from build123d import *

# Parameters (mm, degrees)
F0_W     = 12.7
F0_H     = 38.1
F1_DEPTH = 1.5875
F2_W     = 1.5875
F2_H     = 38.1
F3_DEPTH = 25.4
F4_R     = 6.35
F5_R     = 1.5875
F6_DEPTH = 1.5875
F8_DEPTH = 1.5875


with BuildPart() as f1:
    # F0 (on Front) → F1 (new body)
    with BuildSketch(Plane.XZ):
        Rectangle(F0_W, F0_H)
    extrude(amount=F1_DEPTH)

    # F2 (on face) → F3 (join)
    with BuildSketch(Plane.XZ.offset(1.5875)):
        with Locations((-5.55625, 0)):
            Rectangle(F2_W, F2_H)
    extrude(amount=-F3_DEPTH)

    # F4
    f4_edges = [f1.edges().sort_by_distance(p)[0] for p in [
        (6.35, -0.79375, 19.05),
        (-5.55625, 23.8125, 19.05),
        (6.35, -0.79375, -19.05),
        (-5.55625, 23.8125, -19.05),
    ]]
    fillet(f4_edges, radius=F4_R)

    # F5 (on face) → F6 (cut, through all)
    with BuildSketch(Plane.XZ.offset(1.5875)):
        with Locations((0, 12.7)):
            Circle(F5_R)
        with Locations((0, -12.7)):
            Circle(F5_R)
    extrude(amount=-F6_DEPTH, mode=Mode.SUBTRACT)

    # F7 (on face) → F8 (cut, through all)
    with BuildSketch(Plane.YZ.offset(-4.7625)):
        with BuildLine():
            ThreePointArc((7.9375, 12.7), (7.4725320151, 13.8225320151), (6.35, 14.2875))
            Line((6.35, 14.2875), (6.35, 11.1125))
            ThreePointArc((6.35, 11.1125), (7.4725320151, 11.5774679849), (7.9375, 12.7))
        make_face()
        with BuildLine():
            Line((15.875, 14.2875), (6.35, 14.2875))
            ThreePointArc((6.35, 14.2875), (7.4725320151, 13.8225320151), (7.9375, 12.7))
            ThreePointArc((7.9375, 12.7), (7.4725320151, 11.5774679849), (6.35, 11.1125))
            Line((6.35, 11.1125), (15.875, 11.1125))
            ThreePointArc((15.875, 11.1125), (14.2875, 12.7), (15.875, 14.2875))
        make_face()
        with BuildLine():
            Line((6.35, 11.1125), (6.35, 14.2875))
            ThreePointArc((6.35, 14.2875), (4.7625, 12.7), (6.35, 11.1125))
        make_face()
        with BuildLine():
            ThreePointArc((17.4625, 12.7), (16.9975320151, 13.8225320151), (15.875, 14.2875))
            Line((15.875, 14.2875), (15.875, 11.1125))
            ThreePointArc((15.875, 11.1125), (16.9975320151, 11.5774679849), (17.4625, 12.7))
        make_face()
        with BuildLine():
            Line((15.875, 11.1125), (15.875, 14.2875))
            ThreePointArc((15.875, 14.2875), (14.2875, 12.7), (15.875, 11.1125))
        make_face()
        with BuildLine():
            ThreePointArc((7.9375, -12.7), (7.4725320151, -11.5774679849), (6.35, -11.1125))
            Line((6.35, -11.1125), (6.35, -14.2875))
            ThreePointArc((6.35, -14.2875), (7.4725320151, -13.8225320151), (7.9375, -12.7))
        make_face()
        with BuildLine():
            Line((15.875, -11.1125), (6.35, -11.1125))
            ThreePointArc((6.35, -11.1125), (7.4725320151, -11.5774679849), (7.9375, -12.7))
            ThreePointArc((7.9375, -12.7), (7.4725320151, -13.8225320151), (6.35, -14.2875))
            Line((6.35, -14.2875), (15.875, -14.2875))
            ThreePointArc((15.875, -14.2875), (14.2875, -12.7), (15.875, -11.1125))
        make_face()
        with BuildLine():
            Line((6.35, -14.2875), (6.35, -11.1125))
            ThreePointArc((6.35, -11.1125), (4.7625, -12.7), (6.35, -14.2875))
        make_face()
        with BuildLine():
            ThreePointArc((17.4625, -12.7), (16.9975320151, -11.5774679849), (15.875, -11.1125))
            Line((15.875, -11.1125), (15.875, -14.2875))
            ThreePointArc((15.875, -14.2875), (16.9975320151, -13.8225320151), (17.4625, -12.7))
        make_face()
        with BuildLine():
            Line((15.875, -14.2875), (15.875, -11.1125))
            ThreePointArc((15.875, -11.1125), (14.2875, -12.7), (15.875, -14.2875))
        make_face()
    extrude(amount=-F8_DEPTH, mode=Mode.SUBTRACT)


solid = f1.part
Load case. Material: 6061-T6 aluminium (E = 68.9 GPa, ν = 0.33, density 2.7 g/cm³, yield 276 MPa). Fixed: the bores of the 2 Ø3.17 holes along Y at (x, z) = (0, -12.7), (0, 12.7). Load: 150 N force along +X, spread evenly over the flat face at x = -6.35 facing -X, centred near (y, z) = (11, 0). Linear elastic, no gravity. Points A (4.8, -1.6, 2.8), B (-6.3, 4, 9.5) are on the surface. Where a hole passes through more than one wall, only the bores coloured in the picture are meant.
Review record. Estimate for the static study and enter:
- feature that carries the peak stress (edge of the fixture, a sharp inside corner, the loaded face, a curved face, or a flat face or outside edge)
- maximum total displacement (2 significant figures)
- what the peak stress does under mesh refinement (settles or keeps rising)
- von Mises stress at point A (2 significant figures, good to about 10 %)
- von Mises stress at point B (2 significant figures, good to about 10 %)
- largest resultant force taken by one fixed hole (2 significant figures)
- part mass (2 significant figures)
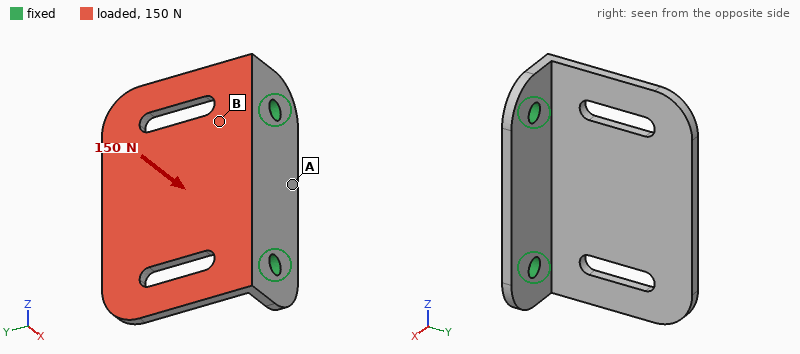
edge of the fixture
0.56 mm
keeps rising
33 MPa
73 MPa
75 N
5.4 g
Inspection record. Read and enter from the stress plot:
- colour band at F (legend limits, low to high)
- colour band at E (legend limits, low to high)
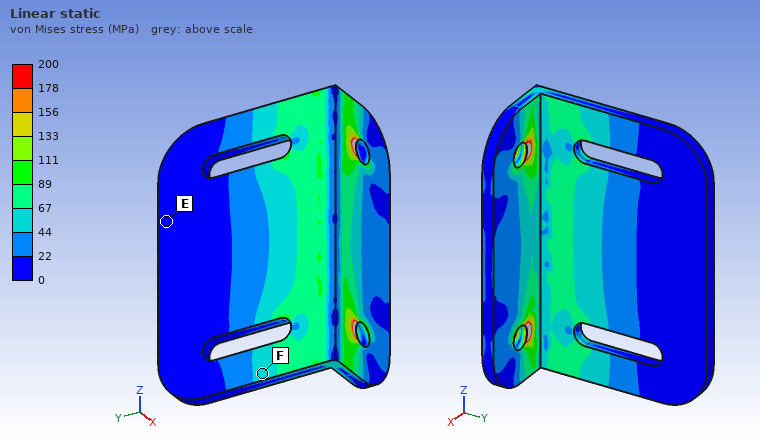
44 to 67 MPa
0 to 22 MPa
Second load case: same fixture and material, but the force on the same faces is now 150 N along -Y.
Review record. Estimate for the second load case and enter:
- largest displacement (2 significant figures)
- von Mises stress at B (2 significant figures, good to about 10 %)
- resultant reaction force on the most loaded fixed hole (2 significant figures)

0.11 mm
9.4 MPa
76 N
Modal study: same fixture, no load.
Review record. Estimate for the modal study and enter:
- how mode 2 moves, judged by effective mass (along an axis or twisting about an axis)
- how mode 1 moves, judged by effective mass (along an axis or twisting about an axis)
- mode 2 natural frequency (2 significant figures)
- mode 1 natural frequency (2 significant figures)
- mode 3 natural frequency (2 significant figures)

twisting about Y
along X
3500 Hz
1700 Hz
8100 Hz
